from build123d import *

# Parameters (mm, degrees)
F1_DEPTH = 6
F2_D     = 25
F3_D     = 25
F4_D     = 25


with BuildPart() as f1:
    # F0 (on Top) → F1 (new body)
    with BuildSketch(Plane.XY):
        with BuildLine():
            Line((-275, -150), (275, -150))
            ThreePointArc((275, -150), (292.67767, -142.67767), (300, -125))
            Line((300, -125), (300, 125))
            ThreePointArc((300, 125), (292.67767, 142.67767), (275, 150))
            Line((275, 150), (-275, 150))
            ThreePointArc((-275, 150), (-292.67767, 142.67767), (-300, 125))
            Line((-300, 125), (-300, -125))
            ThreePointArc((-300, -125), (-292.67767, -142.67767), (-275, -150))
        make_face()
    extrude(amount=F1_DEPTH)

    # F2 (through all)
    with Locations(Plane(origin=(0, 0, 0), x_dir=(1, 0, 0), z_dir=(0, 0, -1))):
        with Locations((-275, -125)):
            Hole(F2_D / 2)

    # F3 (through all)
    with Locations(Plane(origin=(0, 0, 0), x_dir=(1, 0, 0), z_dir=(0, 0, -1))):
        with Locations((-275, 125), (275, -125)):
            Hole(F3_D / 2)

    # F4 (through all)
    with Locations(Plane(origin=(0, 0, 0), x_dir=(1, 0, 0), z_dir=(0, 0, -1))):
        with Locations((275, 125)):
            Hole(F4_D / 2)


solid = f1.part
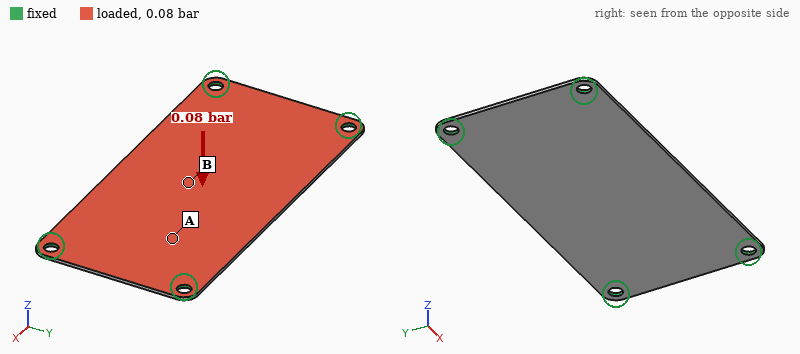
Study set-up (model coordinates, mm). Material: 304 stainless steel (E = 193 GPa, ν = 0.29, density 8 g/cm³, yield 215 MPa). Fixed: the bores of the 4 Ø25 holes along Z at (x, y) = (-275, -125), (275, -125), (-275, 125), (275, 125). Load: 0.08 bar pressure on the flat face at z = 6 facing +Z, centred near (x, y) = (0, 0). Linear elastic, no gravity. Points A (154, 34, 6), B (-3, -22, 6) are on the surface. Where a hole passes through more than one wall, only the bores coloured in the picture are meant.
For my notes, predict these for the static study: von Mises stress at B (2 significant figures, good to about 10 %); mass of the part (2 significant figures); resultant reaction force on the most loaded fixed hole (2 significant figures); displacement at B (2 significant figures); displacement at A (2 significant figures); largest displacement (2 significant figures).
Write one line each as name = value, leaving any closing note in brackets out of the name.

von Mises stress at B = 16 MPa
mass of the part = 8.5 kg
resultant reaction force on the most loaded fixed hole = 360 N
displacement at B = 0.61 mm
displacement at A = 0.33 mm
largest displacement = 0.63 mm
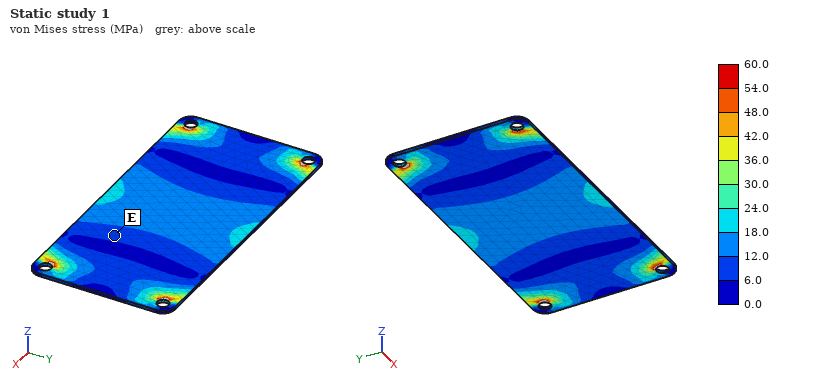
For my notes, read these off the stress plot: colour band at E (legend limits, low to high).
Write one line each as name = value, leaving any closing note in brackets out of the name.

colour band at E = 6.0 to 12.0 MPa
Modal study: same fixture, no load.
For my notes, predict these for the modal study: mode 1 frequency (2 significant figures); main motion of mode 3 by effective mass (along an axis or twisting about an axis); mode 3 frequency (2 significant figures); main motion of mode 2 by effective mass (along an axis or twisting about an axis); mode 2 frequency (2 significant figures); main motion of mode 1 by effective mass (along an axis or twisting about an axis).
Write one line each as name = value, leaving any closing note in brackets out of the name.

mode 1 frequency = 94 Hz
main motion of mode 3 by effective mass = twisting about Y
mode 3 frequency = 260 Hz
main motion of mode 2 by effective mass = twisting about X
mode 2 frequency = 170 Hz
main motion of mode 1 by effective mass = along Z
